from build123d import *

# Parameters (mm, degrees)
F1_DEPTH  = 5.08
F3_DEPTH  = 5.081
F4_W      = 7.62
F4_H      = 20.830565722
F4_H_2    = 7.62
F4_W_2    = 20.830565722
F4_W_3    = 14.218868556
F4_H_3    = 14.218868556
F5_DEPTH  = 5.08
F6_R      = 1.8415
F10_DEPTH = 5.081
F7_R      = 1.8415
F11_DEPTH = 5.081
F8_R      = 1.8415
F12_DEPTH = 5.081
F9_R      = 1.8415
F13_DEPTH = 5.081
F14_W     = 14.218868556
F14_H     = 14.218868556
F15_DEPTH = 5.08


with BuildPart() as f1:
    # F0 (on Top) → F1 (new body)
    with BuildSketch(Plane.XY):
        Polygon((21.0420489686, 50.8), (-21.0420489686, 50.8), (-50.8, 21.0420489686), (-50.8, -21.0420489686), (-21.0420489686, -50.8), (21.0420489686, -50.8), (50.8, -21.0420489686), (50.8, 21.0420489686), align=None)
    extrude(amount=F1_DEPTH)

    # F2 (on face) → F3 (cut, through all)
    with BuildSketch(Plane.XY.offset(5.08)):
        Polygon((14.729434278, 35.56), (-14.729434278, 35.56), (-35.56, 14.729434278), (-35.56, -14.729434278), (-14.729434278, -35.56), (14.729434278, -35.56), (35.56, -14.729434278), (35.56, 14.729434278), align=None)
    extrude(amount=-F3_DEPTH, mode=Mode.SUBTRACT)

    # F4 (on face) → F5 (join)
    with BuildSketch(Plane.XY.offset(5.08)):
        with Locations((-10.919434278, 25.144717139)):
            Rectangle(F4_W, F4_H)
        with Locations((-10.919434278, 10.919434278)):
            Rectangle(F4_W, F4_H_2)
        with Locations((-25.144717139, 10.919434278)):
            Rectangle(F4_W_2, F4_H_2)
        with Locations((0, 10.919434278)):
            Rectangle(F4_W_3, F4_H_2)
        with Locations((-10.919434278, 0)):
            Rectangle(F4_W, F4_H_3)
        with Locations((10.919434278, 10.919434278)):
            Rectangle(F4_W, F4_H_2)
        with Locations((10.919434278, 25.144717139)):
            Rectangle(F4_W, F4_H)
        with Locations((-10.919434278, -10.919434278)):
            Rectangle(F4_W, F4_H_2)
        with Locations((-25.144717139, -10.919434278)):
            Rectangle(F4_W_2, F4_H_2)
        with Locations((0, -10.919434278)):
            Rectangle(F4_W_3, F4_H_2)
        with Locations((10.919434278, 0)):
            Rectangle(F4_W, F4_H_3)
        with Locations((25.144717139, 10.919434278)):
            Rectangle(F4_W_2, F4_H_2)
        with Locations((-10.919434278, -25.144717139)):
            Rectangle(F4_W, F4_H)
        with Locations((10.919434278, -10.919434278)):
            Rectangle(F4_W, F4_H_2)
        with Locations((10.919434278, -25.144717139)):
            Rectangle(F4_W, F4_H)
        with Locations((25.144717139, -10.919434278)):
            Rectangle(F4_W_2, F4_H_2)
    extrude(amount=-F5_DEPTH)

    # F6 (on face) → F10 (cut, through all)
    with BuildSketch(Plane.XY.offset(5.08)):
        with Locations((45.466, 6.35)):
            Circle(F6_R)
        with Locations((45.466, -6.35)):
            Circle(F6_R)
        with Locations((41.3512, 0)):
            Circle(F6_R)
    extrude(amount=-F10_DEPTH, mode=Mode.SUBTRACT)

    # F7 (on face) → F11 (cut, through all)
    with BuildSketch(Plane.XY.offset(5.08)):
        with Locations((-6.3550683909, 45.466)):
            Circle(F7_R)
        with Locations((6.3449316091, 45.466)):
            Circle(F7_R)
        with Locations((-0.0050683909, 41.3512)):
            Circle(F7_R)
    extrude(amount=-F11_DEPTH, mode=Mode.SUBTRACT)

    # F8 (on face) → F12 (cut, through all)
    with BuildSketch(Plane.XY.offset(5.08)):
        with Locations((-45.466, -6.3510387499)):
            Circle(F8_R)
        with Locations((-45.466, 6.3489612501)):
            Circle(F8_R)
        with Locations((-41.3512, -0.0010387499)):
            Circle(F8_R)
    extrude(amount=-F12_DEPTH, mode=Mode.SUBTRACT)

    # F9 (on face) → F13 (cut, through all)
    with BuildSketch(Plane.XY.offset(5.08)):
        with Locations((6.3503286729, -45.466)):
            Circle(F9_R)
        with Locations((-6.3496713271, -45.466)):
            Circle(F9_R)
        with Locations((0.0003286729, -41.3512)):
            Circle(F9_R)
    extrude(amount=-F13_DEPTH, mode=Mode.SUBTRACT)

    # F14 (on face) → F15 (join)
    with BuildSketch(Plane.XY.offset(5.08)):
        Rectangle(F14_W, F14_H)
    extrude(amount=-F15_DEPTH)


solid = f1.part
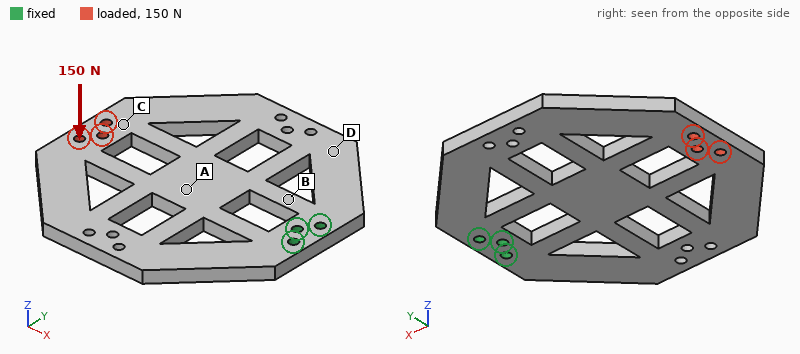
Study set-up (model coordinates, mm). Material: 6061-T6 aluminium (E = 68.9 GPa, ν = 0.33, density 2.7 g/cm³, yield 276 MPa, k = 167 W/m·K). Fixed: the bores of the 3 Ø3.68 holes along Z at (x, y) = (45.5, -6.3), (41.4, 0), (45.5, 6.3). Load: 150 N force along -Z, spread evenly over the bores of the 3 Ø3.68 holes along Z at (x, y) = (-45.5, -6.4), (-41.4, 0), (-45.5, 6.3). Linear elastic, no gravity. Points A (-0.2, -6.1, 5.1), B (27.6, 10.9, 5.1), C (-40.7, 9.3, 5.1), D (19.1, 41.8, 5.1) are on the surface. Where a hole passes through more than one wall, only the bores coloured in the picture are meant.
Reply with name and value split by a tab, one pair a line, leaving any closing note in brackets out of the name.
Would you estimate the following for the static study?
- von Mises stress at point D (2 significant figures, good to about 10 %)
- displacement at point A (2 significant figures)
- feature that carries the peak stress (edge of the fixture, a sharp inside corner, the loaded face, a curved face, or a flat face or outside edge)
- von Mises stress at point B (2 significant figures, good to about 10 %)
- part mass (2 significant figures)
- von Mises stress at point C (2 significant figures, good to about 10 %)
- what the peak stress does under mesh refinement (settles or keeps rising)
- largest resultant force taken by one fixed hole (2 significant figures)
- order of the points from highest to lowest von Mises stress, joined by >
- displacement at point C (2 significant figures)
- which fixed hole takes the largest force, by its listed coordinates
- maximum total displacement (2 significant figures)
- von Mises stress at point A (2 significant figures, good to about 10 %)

von Mises stress at point D	36 MPa
displacement at point A	0.44 mm
feature that carries the peak stress	edge of the fixture
von Mises stress at point B	81 MPa
part mass	87 g
von Mises stress at point C	10 MPa
what the peak stress does under mesh refinement	keeps rising
largest resultant force taken by one fixed hole	500 N
order of the points from highest to lowest von Mises stress, joined by >	B > D > A > C
displacement at point C	1.2 mm
which fixed hole takes the largest force, by its listed coordinates	(41.4, 0)
maximum total displacement	1.4 mm
von Mises stress at point A	22 MPa
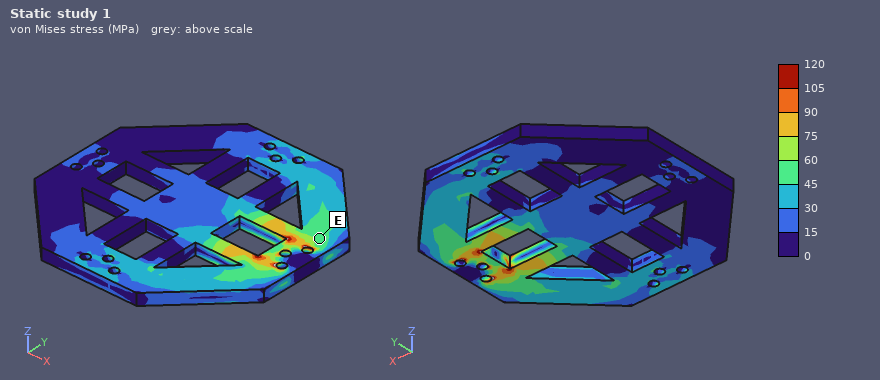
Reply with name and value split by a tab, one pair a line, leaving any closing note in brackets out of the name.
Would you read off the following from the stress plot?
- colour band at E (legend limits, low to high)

colour band at E	45 to 60 MPa
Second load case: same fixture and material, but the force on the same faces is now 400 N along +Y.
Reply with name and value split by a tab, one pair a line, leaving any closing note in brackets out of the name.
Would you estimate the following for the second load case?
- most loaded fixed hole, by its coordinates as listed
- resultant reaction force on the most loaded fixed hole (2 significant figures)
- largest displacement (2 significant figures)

most loaded fixed hole, by its coordinates as listed	(41.4, 0)
resultant reaction force on the most loaded fixed hole	1.9 kN
largest displacement	0.16 mm
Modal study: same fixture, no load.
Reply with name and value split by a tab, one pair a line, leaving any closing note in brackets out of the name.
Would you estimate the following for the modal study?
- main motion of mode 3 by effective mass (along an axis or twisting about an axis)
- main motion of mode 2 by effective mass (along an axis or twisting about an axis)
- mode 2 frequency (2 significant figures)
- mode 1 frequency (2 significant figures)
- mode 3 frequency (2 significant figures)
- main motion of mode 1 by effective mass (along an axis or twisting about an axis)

main motion of mode 3 by effective mass	along Y
main motion of mode 2 by effective mass	twisting about X
mode 2 frequency	730 Hz
mode 1 frequency	360 Hz
mode 3 frequency	1400 Hz
main motion of mode 1 by effective mass	along Z
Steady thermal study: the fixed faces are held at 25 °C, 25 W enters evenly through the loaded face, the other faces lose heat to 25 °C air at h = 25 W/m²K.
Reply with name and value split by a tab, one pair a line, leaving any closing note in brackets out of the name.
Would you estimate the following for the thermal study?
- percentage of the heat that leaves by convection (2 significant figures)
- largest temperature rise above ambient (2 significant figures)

percentage of the heat that leaves by convection	41 %
largest temperature rise above ambient	55 K
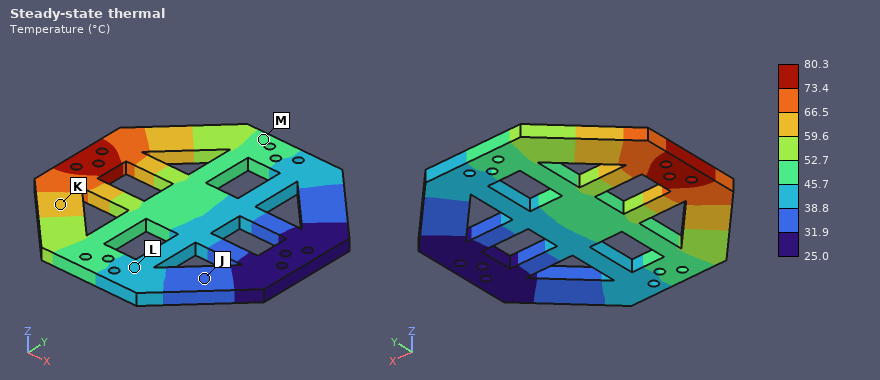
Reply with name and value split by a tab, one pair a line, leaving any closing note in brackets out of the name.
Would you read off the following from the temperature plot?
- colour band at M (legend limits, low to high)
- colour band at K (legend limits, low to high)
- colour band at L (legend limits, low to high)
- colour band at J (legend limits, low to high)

colour band at M	45.7 to 52.7 °C
colour band at K	59.6 to 66.5 °C
colour band at L	38.8 to 45.7 °C
colour band at J	31.9 to 38.8 °C
